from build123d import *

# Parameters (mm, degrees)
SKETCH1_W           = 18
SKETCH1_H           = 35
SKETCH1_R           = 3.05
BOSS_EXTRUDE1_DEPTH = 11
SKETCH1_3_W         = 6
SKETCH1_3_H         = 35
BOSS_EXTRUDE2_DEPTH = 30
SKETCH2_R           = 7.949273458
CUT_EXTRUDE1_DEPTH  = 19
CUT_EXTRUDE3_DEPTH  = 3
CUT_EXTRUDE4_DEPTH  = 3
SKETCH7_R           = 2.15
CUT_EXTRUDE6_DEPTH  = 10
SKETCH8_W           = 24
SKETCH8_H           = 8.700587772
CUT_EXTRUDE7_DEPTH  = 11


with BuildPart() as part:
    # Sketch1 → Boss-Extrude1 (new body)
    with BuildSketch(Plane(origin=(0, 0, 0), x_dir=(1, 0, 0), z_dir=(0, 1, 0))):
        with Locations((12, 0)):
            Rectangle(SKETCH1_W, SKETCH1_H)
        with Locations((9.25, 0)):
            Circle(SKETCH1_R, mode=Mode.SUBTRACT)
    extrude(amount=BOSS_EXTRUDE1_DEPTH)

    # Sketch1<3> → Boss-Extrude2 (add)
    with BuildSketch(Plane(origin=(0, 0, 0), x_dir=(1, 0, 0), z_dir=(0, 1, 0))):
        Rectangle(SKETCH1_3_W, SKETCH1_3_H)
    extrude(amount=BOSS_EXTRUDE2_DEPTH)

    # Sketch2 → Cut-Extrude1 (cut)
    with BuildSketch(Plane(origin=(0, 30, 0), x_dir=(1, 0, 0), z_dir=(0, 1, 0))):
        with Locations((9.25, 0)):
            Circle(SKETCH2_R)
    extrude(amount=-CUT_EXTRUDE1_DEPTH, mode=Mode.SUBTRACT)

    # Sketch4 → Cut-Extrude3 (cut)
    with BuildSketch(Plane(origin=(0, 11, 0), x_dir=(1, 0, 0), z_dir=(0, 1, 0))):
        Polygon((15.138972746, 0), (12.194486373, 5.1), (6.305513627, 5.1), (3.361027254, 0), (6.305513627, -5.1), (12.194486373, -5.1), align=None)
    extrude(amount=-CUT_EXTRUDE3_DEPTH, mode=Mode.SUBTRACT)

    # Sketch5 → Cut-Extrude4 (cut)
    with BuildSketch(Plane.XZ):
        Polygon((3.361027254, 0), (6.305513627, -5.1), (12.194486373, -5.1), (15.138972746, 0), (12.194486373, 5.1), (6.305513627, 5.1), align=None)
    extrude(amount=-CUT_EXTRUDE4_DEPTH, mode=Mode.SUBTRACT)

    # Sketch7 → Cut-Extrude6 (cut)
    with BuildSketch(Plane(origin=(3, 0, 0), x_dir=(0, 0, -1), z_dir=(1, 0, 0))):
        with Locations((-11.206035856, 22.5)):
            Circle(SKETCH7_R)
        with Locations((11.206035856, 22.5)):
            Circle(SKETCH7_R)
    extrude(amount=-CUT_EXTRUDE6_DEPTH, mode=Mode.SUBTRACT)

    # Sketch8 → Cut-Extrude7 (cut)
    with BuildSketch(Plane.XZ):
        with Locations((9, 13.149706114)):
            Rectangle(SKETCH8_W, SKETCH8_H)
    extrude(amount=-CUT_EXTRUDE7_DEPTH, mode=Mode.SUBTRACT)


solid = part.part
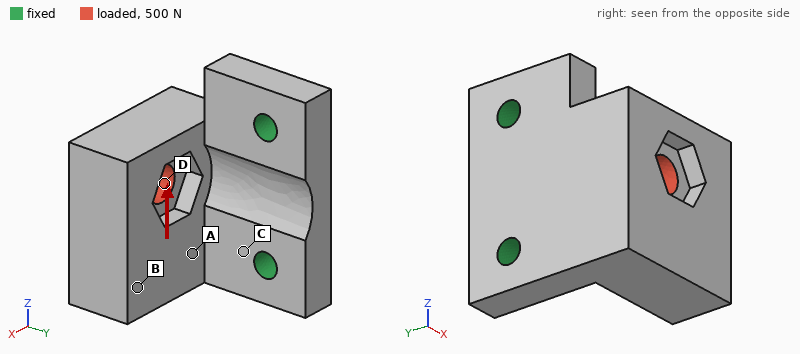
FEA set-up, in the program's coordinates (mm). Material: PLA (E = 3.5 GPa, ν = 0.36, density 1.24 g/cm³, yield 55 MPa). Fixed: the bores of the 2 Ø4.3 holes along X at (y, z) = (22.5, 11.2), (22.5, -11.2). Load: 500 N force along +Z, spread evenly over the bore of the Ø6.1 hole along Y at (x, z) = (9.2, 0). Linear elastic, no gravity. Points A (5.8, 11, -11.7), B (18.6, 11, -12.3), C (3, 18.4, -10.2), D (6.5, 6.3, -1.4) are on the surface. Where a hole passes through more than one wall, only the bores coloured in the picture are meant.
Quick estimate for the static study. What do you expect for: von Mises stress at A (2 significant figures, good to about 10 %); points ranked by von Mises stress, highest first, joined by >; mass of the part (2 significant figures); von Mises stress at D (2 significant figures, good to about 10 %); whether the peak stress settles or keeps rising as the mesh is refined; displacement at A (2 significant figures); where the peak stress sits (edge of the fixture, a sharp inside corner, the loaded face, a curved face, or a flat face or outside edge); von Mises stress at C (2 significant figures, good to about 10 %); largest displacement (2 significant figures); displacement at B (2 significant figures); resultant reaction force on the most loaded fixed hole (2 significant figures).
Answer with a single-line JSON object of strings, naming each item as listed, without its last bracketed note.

{"von Mises stress at A": "8.4 MPa", "points ranked by von Mises stress, highest first, joined by >": "C > D > A > B", "mass of the part": "12 g", "von Mises stress at D": "13 MPa", "whether the peak stress settles or keeps rising as the mesh is refined": "keeps rising", "displacement at A": "0.14 mm", "where the peak stress sits": "a sharp inside corner", "von Mises stress at C": "16 MPa", "largest displacement": "0.35 mm", "displacement at B": "0.29 mm", "resultant reaction force on the most loaded fixed hole": "450 N"}
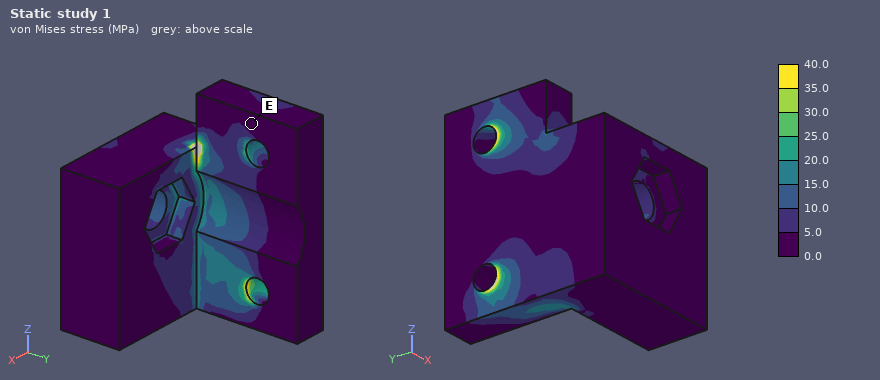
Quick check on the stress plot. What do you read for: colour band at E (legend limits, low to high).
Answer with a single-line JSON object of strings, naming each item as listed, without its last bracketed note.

{"colour band at E": "0.0 to 5.0 MPa"}
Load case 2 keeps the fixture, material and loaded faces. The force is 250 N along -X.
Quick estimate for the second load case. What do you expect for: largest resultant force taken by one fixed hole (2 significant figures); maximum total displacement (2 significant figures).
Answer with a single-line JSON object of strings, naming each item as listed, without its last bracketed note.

{"largest resultant force taken by one fixed hole": "130 N", "maximum total displacement": "0.59 mm"}
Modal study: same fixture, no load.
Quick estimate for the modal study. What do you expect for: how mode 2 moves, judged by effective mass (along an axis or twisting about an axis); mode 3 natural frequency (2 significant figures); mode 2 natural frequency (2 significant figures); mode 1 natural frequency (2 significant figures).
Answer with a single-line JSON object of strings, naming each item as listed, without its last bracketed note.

{"how mode 2 moves, judged by effective mass": "along Z", "mode 3 natural frequency": "4400 Hz", "mode 2 natural frequency": "2400 Hz", "mode 1 natural frequency": "1200 Hz"}
